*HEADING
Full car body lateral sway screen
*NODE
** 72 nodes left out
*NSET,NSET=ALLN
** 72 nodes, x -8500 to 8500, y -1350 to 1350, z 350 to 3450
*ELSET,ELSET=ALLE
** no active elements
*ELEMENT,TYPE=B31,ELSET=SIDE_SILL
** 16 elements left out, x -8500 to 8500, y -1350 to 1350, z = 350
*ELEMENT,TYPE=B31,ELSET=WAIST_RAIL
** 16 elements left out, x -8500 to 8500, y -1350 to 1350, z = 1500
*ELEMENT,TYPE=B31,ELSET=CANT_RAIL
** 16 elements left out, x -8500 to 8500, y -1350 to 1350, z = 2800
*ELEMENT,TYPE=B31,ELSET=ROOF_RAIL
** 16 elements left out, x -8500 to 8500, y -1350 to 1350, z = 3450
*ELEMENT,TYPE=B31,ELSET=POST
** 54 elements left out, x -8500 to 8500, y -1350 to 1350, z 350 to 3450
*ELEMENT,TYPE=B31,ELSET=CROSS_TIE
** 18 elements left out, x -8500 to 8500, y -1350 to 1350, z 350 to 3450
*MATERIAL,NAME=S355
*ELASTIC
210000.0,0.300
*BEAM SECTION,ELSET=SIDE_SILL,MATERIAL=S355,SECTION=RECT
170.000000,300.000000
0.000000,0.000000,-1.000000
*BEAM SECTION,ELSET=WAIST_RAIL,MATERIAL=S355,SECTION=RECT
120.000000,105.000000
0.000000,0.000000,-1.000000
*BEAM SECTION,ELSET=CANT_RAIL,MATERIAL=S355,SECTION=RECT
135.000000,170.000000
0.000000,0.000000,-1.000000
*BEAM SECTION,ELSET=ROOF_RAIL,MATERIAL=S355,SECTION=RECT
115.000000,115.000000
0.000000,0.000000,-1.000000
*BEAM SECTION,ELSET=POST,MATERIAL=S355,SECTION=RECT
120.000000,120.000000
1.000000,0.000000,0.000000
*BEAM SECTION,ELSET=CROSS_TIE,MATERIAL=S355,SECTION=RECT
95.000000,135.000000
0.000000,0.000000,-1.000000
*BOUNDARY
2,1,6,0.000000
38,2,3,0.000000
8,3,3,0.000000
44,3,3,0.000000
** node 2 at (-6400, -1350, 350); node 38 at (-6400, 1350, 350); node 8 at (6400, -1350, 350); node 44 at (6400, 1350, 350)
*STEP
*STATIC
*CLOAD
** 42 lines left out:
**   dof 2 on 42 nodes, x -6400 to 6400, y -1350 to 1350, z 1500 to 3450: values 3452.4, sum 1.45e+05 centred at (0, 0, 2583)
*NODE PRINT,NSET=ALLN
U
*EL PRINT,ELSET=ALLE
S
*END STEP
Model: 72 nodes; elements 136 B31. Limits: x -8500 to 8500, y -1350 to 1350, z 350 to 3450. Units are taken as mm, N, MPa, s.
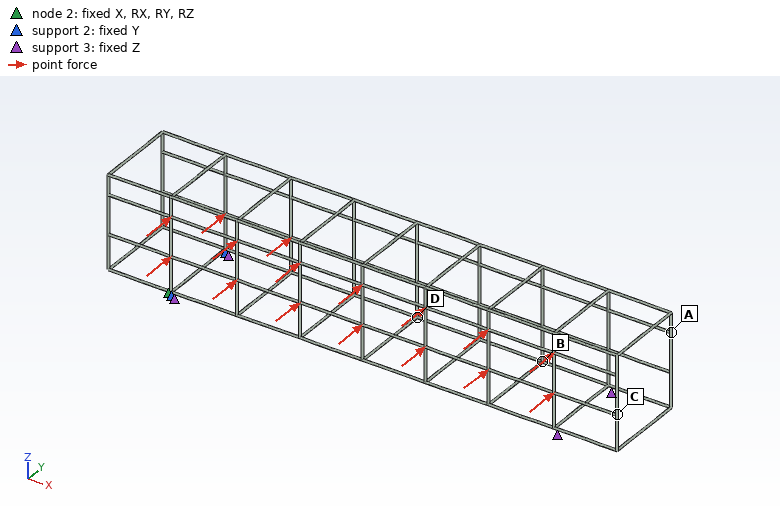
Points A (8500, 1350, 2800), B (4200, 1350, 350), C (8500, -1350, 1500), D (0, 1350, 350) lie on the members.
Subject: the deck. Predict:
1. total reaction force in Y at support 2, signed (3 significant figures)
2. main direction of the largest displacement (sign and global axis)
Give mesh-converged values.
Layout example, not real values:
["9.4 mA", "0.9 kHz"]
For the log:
["-1.45e+05 N", "+Y"]
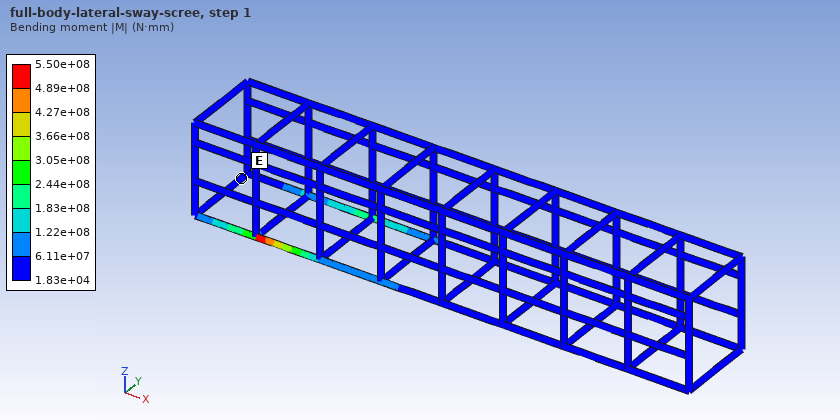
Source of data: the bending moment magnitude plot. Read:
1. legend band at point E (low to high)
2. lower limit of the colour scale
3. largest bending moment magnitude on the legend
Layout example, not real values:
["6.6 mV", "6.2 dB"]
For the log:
["1.83e+04 to 6.11e+07 N·mm", "1.83e+04 N·mm", "5.50e+08 N·mm"]
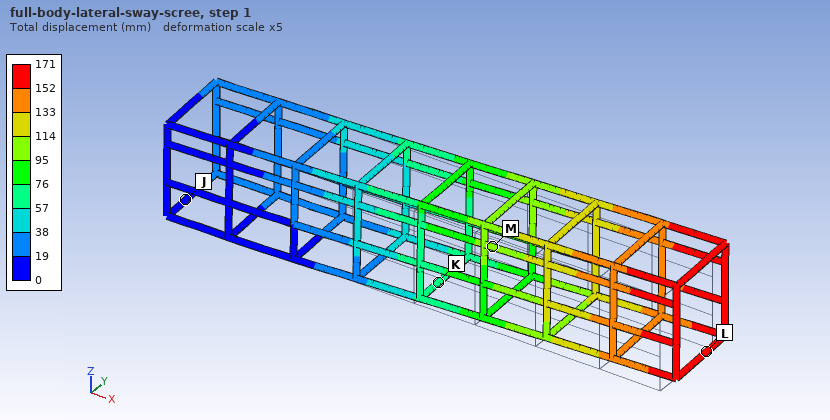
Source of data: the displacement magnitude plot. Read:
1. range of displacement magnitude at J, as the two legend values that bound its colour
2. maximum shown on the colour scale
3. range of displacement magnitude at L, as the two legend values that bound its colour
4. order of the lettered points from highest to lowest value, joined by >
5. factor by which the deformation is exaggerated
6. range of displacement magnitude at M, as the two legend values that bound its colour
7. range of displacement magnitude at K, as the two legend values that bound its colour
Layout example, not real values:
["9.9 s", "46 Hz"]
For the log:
["0 to 19 mm", "171 mm", "152 to 171 mm", "L > M > K > J", "5", "95 to 114 mm", "57 to 76 mm"]
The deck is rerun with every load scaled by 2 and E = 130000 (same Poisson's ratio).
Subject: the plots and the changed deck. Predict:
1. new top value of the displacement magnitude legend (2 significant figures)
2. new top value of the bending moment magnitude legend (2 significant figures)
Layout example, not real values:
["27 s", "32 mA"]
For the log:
["550 mm", "1.1e+09 N·mm"]
